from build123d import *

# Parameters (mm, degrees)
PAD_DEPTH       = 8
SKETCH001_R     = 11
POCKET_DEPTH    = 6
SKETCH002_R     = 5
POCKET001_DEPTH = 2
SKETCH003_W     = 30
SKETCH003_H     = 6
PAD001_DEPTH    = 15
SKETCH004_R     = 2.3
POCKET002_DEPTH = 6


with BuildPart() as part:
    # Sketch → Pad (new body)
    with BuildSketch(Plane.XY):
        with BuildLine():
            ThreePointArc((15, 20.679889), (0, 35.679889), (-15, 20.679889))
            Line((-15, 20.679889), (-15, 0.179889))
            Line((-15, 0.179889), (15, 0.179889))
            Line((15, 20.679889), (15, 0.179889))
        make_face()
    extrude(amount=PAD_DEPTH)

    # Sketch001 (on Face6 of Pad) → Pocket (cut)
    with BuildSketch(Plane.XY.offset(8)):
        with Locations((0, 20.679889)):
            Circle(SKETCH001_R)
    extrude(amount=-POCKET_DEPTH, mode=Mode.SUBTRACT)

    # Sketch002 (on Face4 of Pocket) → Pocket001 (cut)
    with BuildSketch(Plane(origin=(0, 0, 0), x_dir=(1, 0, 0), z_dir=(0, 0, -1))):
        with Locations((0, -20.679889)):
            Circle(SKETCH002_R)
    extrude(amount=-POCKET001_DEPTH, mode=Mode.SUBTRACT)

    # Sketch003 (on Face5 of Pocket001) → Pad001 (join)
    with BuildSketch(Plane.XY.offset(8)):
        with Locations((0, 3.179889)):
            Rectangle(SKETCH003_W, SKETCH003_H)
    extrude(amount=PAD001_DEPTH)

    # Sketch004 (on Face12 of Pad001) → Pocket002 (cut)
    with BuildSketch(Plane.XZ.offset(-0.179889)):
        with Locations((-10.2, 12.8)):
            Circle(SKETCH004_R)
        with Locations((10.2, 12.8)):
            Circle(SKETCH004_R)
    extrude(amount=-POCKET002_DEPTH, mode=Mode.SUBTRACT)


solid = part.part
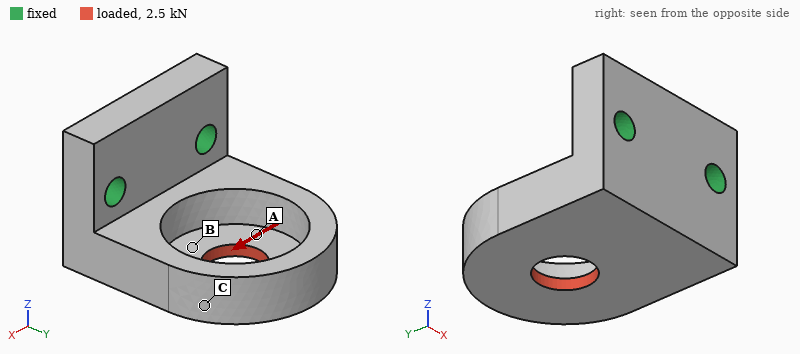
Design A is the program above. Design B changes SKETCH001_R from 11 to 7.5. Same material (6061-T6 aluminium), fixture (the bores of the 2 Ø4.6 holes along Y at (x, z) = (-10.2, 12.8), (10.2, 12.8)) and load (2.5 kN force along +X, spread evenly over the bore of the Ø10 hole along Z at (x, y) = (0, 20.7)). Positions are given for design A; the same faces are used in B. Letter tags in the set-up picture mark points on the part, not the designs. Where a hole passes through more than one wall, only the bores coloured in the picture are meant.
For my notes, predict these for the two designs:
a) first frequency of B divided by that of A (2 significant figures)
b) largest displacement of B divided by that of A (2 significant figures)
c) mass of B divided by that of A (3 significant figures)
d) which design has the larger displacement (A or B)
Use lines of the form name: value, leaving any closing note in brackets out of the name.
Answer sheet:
first frequency of B divided by that of A: 0.95
largest displacement of B divided by that of A: 0.65
mass of B divided by that of A: 1.16
which design has the larger displacement: A
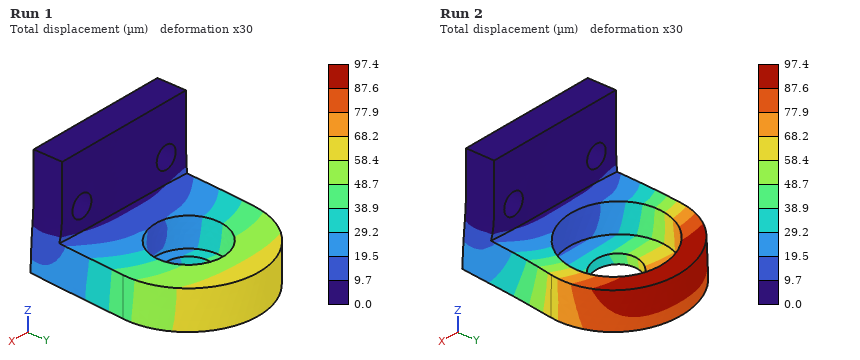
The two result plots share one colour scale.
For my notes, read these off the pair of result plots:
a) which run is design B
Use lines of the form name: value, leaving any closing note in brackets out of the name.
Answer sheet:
which run is design B: Run 1
